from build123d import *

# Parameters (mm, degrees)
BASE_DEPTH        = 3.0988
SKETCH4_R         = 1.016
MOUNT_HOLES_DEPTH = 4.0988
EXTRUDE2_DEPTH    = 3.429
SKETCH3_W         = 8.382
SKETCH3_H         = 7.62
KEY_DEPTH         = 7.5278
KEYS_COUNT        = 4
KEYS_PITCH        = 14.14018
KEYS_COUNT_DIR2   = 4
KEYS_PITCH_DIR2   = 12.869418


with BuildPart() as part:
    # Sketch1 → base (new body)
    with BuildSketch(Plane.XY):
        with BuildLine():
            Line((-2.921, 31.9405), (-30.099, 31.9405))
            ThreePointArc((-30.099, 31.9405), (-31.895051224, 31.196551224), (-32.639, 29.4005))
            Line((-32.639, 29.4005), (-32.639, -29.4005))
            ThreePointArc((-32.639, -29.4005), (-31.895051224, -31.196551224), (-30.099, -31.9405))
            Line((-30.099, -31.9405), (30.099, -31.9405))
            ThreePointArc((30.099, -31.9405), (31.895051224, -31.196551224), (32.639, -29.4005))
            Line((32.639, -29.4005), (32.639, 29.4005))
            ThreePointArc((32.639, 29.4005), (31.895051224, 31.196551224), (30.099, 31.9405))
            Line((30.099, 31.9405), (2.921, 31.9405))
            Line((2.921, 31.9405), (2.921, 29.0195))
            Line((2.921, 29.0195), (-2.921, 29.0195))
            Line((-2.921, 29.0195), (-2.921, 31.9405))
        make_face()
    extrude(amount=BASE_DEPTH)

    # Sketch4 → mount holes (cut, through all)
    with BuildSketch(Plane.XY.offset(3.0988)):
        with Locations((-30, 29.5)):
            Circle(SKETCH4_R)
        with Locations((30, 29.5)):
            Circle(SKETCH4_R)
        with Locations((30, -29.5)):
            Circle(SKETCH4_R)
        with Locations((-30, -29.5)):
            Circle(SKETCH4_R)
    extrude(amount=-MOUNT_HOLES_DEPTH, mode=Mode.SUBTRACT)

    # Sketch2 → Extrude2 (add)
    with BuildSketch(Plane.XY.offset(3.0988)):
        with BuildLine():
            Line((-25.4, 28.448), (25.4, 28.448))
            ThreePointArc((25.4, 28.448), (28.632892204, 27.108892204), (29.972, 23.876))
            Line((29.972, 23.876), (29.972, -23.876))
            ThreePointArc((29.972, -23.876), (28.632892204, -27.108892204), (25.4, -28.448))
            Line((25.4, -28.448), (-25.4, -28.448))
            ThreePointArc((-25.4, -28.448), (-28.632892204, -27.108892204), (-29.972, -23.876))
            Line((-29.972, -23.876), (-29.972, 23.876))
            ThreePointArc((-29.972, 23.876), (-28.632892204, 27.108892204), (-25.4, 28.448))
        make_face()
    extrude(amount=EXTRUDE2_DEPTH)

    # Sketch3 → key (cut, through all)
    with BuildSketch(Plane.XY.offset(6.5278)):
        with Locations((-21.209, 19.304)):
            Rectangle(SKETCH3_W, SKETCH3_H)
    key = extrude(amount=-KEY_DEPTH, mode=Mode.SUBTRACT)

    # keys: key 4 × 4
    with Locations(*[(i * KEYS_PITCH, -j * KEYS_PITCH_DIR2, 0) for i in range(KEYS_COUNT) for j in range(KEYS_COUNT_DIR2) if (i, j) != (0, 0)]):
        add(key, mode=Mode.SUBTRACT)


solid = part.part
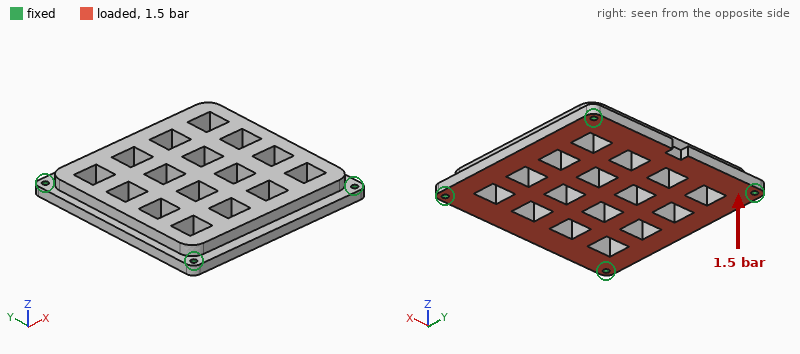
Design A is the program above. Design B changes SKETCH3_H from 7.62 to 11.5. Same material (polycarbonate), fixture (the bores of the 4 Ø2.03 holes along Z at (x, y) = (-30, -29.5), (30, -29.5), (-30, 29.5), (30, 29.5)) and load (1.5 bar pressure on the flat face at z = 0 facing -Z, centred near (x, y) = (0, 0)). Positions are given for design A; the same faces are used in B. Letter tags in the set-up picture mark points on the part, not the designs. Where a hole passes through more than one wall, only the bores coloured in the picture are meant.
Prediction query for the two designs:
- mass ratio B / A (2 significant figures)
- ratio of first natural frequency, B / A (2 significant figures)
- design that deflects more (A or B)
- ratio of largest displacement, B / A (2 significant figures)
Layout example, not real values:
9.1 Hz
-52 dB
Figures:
0.81
0.96
B
1.1
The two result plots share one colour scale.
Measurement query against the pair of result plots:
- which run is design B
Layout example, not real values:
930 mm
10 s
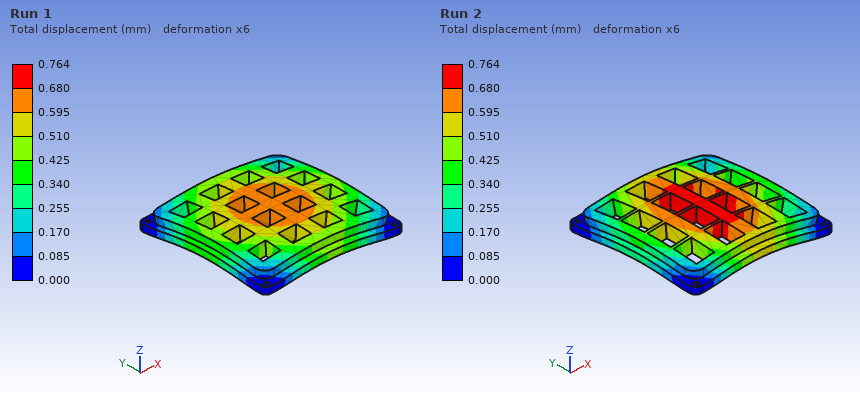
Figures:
Run 2
